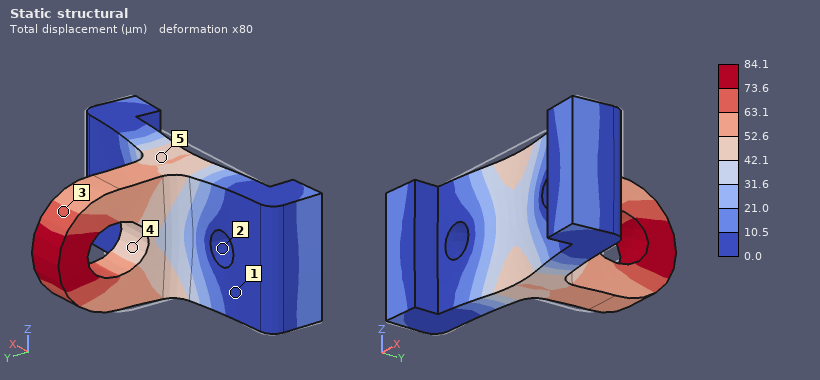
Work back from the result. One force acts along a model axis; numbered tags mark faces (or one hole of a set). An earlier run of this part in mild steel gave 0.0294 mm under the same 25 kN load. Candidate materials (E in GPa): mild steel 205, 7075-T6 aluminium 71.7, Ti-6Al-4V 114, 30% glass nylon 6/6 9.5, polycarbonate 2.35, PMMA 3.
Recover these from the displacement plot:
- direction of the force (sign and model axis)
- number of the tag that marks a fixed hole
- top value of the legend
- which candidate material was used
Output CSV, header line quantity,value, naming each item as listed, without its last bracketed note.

quantity,value
direction of the force,+Y
number of the tag that marks a fixed hole,2
top value of the legend,84.1 µm
which candidate material was used,7075-T6 aluminium
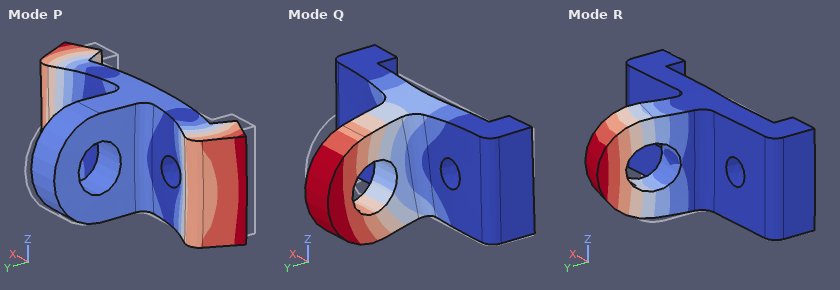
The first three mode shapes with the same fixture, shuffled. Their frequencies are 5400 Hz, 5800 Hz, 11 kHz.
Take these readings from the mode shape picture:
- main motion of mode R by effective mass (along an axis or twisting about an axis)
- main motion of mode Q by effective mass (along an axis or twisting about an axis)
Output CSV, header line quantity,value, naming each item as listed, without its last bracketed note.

quantity,value
main motion of mode R by effective mass,along X
main motion of mode Q by effective mass,along Z
